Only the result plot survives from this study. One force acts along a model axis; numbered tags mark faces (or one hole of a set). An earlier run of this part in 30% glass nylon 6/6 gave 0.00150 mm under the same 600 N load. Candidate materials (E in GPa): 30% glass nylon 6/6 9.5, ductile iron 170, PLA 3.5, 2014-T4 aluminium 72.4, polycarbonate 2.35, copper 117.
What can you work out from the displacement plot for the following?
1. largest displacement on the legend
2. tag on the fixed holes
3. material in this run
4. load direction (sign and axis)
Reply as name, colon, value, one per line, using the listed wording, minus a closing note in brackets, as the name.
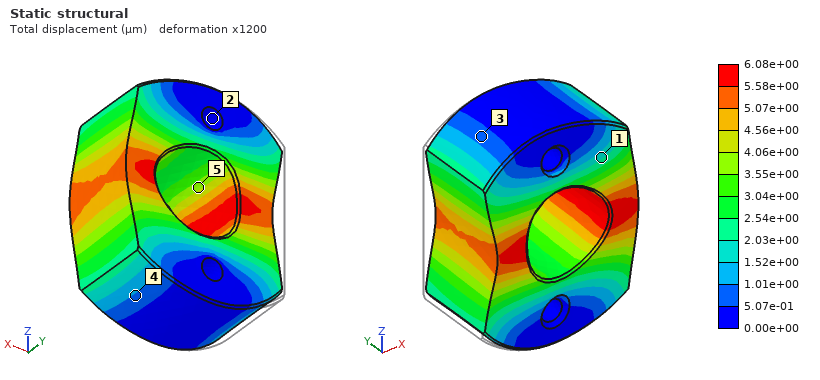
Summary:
largest displacement on the legend: 6.08e+00 µm
tag on the fixed holes: 2
material in this run: polycarbonate
load direction: +X
